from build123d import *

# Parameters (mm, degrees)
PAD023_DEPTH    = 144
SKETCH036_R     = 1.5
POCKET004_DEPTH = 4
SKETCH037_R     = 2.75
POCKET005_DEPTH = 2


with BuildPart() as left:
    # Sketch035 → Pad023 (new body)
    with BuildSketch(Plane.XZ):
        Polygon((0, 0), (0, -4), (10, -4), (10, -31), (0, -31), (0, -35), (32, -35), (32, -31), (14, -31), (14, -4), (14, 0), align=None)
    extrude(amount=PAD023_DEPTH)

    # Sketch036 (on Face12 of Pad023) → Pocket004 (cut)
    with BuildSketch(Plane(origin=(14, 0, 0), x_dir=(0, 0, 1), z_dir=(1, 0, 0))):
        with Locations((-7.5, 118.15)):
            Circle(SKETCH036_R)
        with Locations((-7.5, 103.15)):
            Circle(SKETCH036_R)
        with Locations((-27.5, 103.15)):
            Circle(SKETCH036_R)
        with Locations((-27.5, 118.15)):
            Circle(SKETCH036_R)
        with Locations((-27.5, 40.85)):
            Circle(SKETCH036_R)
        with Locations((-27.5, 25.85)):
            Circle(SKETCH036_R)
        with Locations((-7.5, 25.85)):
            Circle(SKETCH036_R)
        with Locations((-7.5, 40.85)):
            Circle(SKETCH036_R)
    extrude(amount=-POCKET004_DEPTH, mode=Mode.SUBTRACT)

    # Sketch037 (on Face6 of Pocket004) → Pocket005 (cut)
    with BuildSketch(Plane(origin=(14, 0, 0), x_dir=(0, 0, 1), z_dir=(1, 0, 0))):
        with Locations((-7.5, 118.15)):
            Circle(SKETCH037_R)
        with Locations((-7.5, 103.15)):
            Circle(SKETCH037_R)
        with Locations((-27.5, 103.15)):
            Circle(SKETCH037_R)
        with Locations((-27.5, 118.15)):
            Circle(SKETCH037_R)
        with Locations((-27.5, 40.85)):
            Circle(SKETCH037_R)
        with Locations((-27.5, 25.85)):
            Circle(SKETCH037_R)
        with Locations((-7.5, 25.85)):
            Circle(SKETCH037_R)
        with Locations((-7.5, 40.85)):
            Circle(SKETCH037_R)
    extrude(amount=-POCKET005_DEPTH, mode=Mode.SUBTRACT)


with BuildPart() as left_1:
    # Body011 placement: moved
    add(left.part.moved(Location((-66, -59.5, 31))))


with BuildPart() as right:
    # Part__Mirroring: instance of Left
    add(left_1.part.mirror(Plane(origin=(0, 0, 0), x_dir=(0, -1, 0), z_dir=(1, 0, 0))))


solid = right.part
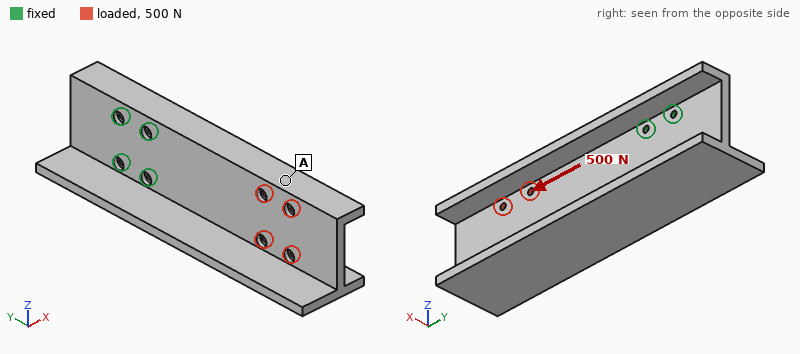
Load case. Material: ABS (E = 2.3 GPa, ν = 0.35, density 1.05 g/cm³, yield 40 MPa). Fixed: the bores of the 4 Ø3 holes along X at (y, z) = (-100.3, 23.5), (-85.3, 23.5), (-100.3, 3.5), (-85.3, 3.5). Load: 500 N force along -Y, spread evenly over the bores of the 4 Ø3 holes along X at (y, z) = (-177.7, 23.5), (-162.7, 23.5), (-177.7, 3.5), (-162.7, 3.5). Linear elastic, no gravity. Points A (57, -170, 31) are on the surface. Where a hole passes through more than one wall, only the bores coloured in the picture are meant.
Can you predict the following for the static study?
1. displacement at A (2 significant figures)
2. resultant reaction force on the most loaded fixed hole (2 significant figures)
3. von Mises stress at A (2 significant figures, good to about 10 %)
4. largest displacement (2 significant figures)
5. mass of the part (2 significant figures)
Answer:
0.11 mm
170 N
1.5 MPa
0.23 mm
44 g
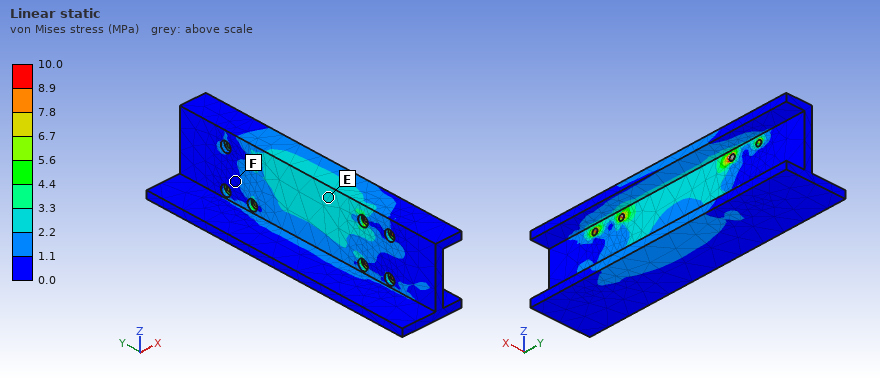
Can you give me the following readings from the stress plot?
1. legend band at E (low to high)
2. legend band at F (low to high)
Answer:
2.2 to 3.3 MPa
0.0 to 1.1 MPa
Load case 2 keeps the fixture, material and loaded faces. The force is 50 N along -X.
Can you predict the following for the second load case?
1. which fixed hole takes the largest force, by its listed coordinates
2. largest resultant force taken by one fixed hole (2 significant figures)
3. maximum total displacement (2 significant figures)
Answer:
(-100.3, 3.5)
160 N
1.6 mm
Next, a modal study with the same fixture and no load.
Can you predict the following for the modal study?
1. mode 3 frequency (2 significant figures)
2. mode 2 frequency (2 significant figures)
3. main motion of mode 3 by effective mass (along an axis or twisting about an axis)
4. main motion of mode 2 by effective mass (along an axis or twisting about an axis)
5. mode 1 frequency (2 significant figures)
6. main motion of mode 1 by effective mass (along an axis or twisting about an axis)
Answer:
610 Hz
420 Hz
along Z
twisting about Y
250 Hz
along X
